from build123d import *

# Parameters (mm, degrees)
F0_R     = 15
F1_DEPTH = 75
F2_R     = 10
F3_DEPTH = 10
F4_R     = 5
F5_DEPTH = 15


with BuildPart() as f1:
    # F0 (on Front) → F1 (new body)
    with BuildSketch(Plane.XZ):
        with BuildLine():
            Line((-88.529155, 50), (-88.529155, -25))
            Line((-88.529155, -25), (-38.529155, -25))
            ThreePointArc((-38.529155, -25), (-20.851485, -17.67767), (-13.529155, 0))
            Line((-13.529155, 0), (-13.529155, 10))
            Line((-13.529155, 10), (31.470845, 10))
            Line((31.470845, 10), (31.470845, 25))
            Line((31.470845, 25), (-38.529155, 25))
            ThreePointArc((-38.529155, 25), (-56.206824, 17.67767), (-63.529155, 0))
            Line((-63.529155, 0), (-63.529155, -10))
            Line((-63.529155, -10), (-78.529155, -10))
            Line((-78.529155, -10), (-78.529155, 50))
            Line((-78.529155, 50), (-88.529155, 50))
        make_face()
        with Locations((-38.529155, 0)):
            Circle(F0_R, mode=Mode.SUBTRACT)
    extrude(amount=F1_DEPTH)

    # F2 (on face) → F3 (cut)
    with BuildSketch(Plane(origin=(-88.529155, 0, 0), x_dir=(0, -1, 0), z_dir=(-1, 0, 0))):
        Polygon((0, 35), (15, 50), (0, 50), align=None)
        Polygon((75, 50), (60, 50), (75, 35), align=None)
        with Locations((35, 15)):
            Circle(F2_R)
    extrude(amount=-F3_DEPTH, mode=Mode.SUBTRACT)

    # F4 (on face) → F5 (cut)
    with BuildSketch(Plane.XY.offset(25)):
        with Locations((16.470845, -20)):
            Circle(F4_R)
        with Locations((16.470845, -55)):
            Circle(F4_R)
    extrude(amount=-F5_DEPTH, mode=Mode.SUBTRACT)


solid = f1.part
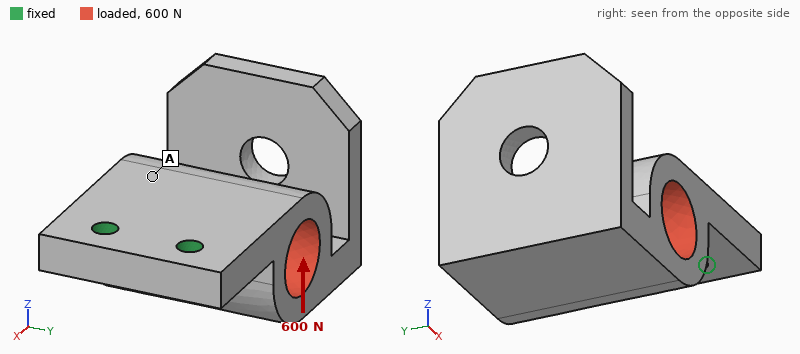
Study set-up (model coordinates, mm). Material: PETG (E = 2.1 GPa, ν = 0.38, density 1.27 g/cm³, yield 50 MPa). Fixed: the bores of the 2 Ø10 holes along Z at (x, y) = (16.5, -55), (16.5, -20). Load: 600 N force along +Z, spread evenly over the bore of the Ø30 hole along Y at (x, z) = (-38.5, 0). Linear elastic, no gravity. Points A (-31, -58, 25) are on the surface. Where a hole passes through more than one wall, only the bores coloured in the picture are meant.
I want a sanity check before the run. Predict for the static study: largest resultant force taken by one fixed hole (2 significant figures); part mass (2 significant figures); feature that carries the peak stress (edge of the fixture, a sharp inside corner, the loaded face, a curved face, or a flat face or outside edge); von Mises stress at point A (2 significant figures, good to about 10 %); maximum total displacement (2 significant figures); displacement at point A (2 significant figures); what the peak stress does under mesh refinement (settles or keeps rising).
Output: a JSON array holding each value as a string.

["300 N", "290 g", "edge of the fixture", "2.0 MPa", "1.8 mm", "0.59 mm", "keeps rising"]
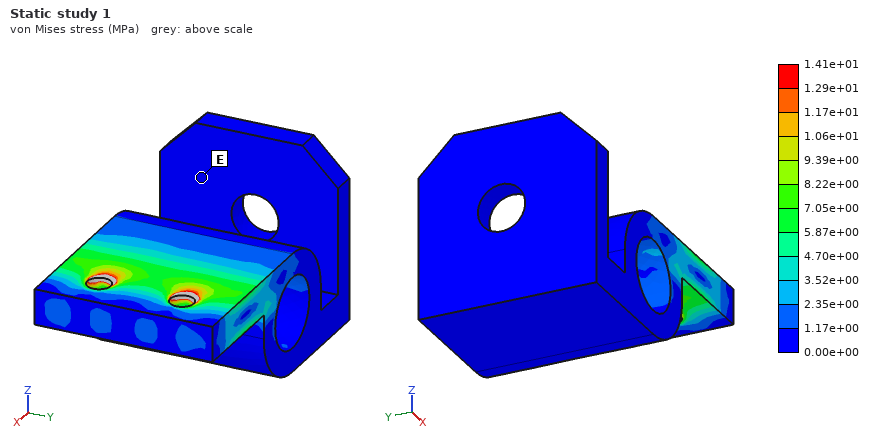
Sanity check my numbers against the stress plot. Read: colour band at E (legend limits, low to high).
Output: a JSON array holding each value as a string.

["0.00e+00 to 1.17e+00 MPa"]
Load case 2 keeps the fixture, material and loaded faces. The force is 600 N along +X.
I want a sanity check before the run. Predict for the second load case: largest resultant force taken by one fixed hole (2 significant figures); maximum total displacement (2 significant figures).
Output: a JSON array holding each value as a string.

["300 N", "0.87 mm"]
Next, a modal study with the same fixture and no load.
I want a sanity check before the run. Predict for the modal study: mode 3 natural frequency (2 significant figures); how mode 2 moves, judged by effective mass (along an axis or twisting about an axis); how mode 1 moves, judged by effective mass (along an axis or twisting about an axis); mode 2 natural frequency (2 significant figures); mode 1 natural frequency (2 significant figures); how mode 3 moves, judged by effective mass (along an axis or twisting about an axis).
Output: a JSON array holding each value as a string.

["480 Hz", "along X", "along Z", "430 Hz", "180 Hz", "along Y"]
